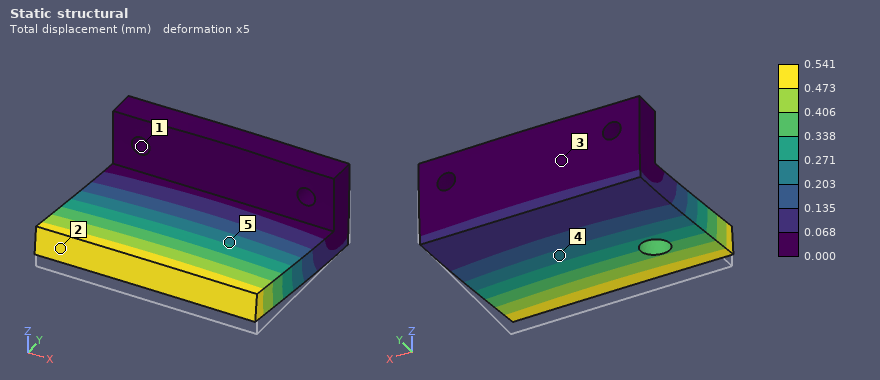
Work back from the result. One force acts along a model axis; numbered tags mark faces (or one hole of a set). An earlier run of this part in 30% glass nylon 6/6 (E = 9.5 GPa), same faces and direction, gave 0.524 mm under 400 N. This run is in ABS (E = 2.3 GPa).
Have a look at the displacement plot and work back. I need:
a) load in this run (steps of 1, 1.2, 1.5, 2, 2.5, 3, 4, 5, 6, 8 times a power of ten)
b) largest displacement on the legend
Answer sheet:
100 N
0.541 mm
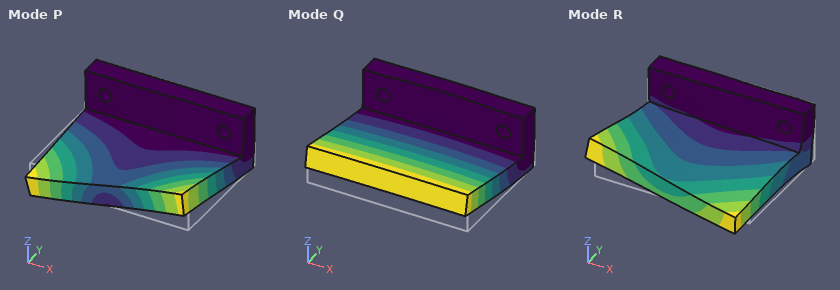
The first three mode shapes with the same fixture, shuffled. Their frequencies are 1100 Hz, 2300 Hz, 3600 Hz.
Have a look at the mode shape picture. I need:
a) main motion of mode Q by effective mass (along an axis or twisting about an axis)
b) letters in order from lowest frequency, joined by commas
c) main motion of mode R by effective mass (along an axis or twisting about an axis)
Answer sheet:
along Z
Q, P, R
along X
